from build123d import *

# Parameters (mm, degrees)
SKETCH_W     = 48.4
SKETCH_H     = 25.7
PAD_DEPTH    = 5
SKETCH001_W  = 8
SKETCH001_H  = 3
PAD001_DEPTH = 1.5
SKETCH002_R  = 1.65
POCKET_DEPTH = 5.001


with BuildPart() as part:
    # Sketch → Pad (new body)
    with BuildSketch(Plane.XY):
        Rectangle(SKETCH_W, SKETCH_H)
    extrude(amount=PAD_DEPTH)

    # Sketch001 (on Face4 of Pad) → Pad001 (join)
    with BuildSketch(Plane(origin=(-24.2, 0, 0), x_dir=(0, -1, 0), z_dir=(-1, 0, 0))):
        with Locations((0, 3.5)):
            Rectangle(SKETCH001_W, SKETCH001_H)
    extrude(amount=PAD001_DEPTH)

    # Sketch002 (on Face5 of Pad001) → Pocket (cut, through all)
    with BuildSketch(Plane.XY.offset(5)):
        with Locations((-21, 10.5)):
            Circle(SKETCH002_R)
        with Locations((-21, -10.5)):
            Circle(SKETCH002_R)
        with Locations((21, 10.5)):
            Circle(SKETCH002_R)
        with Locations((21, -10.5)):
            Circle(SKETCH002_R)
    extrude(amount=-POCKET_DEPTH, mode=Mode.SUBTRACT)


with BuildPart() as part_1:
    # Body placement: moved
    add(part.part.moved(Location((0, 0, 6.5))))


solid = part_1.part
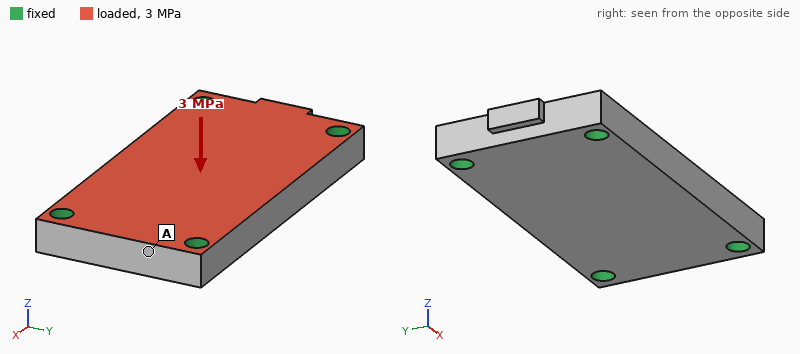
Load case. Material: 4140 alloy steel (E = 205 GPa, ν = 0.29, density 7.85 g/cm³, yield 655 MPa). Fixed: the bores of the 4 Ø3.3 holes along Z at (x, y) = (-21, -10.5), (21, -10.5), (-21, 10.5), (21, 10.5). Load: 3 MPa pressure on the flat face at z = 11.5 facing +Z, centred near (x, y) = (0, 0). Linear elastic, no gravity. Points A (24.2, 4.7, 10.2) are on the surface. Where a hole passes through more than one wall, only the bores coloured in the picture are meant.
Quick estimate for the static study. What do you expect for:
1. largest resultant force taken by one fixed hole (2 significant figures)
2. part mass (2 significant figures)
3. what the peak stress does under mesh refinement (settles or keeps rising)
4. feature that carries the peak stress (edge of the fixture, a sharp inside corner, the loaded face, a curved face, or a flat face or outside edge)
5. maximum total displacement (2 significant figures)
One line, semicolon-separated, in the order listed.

930 N; 48 g; keeps rising; edge of the fixture; 15 µm
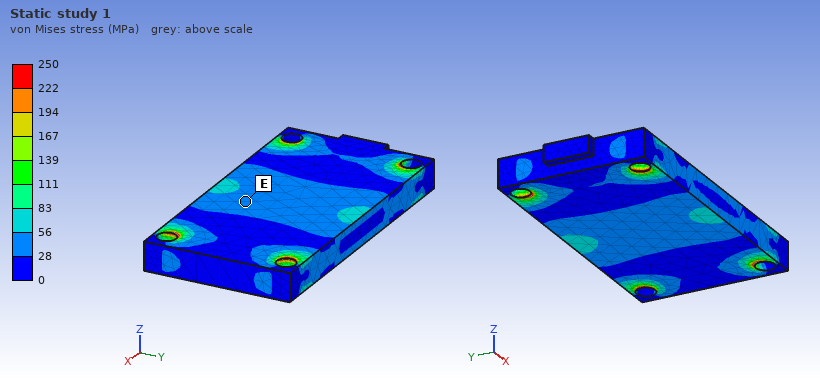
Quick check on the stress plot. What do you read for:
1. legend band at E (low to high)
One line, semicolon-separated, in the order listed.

28 to 56 MPa
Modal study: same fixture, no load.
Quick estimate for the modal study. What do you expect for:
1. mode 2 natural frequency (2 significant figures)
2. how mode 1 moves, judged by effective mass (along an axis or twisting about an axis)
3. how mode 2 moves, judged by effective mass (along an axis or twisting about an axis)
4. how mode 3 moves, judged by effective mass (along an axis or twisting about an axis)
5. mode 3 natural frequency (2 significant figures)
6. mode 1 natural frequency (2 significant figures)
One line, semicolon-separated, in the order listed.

20 kHz; along Z; twisting about X; twisting about Y; 32 kHz; 13 kHz
